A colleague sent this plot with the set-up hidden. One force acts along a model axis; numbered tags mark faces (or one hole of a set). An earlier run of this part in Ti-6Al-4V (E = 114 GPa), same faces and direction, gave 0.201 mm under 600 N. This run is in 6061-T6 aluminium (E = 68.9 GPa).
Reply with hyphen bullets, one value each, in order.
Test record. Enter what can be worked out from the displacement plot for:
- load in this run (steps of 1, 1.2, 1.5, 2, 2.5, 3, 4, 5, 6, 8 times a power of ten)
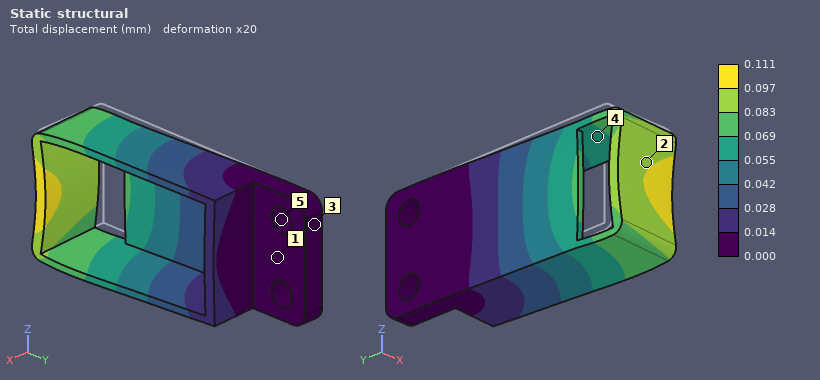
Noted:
- 200 N
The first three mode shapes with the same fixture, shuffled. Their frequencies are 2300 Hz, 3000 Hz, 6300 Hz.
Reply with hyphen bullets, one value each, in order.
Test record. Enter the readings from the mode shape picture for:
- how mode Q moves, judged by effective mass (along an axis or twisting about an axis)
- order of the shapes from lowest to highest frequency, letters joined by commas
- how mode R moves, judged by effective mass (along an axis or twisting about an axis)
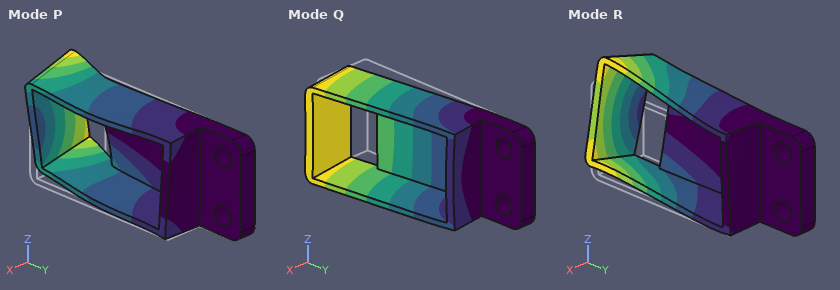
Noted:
- along X
- Q, R, P
- along Z
